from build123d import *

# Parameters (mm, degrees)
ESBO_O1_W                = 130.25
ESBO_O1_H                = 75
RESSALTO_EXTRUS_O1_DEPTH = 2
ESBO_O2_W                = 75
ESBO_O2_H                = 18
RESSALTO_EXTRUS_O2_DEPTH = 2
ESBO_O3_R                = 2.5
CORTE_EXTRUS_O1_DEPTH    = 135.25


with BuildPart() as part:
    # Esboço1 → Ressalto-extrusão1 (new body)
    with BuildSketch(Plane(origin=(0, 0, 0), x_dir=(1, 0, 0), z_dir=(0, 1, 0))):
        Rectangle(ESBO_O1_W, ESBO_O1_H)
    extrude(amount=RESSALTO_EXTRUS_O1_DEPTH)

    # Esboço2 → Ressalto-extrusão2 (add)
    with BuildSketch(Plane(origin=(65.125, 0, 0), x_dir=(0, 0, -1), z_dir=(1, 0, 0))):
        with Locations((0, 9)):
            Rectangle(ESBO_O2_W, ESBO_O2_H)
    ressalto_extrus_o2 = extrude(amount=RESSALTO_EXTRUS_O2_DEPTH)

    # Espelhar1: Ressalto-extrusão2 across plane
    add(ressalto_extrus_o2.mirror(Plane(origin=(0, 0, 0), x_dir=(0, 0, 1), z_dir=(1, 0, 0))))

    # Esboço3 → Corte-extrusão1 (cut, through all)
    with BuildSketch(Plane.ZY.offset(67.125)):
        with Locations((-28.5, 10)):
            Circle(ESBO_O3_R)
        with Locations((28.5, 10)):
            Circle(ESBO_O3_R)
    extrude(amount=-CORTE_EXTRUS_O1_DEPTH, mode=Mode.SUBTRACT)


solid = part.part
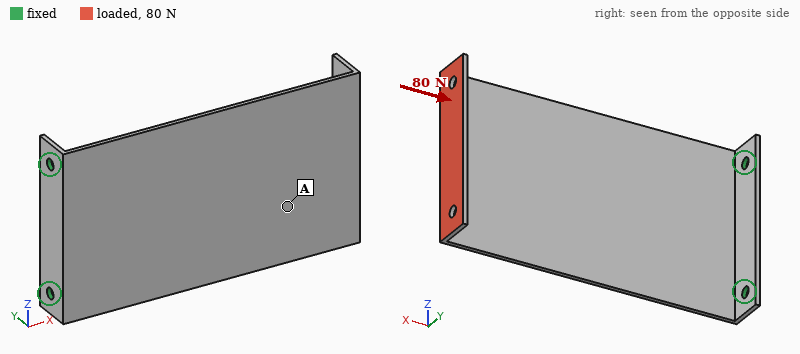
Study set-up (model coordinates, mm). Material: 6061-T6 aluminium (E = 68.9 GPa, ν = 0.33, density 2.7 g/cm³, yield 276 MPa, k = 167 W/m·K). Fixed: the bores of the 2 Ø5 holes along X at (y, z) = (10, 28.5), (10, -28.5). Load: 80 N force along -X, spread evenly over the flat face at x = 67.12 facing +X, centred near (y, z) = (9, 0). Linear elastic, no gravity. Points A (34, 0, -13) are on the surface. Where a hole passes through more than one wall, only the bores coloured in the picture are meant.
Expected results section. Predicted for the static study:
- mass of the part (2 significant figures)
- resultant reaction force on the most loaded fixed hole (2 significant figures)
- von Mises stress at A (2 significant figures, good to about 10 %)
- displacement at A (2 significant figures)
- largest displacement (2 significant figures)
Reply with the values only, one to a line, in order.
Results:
67 g
41 N
11 MPa
0.98 mm
1.7 mm
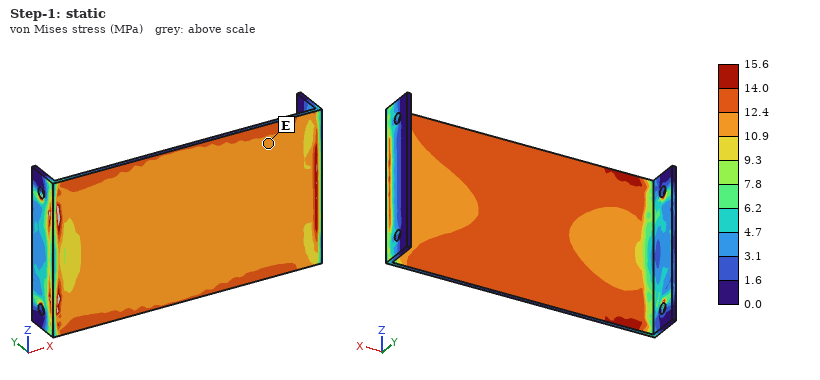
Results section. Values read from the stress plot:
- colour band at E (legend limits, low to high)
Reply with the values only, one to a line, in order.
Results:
10.9 to 12.4 MPa
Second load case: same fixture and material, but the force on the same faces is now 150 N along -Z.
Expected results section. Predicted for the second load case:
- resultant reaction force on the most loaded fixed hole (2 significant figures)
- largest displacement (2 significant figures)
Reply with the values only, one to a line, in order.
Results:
350 N
1.4 mm
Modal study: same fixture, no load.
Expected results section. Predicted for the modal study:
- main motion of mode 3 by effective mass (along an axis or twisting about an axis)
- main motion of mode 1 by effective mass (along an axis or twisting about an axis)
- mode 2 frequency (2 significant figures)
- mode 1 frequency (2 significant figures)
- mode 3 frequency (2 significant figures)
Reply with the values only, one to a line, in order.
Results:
along Y
along Y
300 Hz
69 Hz
450 Hz
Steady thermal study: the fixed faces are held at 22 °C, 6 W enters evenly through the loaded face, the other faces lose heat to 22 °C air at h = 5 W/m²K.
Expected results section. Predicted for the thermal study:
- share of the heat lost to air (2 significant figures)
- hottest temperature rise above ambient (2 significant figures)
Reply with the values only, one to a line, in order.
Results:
29 %
30 K
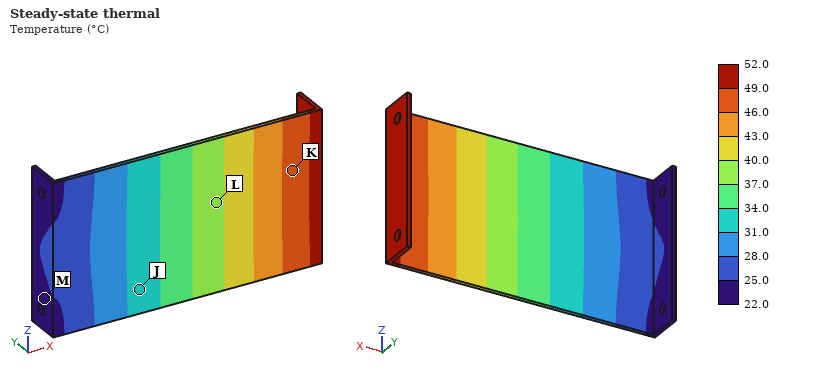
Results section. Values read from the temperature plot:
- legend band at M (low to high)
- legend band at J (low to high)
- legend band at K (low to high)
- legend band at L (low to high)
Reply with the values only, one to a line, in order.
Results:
22.0 to 25.0 °C
31.0 to 34.0 °C
46.0 to 49.0 °C
37.0 to 40.0 °C
